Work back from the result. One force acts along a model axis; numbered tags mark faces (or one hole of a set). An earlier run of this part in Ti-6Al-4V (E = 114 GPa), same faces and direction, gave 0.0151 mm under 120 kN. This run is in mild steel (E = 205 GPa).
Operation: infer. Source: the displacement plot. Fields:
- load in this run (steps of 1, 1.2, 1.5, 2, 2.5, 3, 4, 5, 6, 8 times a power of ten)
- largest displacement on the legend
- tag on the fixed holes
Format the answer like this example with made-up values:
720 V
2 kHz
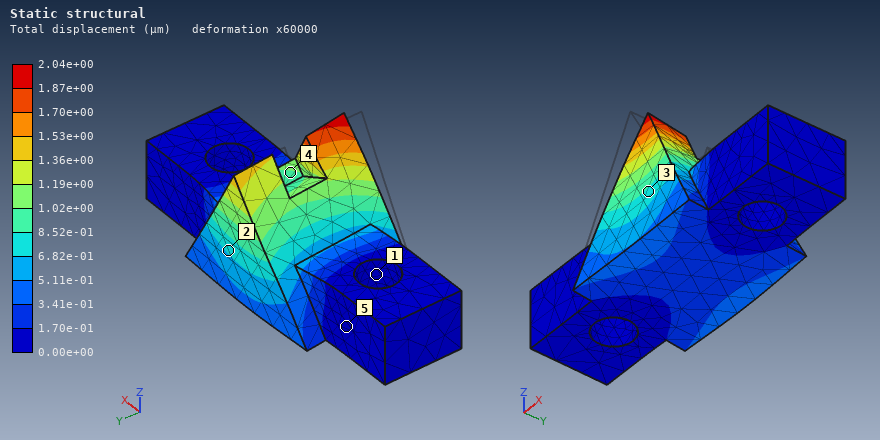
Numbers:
30 kN
2.04e+00 µm
1
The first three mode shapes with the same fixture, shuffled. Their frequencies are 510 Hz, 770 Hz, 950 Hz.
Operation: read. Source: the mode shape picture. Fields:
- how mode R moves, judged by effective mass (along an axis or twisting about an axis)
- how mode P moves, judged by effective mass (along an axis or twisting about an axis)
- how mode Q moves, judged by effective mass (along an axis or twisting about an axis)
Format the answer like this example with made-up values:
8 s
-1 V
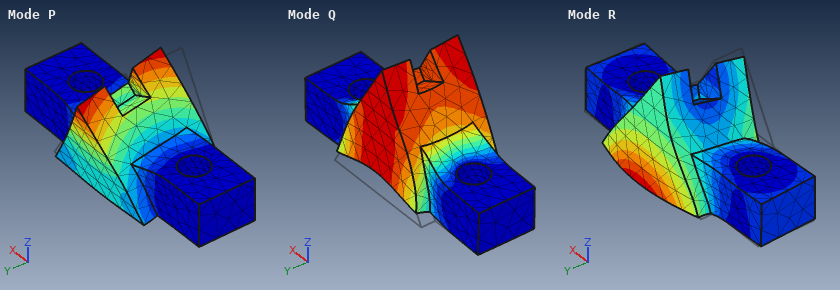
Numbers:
along Y
along Y
along Z
